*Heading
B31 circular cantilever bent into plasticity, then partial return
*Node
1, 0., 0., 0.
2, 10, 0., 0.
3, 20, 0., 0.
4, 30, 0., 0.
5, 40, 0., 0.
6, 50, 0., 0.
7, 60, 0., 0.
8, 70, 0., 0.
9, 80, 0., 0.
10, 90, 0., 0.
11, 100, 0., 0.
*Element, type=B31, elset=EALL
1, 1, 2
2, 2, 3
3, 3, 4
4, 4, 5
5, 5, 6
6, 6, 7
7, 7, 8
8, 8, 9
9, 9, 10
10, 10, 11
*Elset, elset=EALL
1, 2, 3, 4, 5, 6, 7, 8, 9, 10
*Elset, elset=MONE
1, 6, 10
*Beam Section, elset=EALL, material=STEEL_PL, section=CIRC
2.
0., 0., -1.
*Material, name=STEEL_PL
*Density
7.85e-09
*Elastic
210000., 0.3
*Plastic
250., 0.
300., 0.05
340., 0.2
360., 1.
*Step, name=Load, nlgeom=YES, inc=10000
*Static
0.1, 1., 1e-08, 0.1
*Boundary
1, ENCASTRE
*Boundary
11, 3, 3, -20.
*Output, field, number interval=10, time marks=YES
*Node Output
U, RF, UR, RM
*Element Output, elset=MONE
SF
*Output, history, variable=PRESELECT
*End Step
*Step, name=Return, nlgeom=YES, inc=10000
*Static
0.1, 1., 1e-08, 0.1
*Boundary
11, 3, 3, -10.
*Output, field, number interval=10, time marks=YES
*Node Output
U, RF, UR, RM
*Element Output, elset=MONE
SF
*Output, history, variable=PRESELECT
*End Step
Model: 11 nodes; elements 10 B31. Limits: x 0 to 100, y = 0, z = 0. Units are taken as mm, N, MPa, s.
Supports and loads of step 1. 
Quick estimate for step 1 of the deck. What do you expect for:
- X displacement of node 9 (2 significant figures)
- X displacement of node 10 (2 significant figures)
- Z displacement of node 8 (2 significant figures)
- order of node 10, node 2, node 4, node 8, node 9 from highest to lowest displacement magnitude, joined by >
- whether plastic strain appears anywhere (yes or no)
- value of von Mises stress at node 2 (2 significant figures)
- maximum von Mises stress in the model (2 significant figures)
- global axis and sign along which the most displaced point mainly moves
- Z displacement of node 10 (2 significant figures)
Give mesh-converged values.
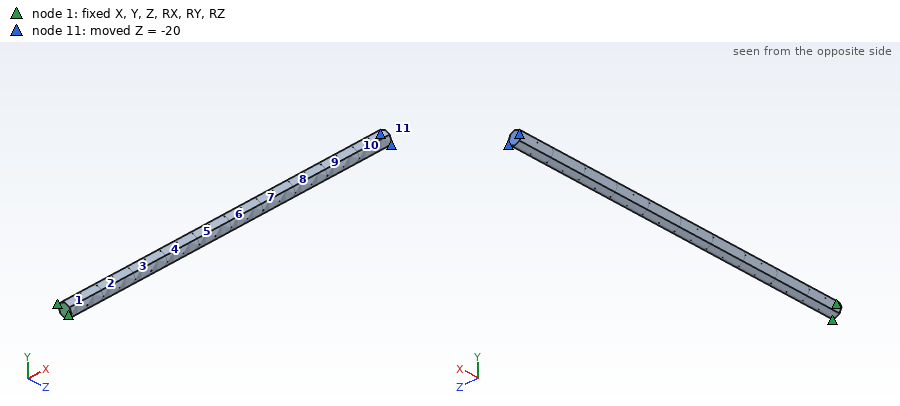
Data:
-1.3 mm
-1.6 mm
-13 mm
node 10 > node 9 > node 8 > node 4 > node 2
yes
380 MPa
420 MPa
-Z
-18 mm
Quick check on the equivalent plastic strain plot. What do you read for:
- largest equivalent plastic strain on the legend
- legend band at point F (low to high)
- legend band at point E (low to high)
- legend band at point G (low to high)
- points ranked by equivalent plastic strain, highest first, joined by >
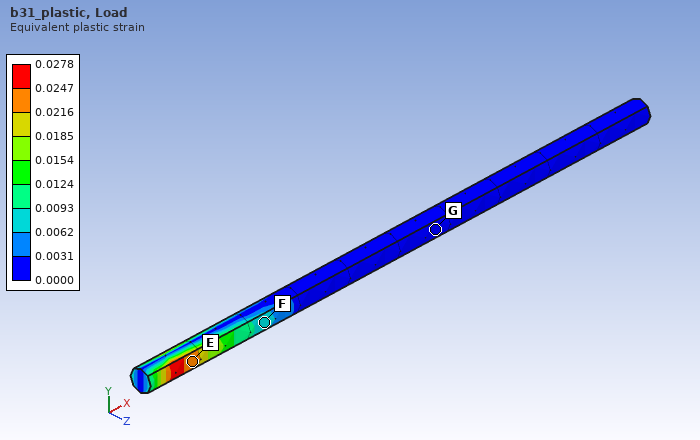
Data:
0.0278
0.0062 to 0.0093
0.0216 to 0.0247
0.0000 to 0.0031
E > F > G
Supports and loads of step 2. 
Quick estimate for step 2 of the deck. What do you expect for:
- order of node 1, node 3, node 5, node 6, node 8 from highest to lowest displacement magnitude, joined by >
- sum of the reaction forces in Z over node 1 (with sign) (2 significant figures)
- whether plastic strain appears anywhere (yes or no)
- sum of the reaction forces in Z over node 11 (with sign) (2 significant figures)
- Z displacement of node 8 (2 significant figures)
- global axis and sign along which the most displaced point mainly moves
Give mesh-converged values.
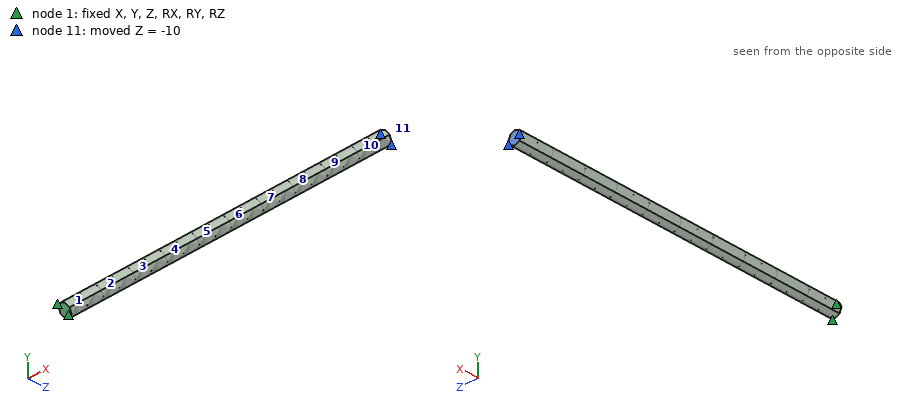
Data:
node 8 > node 6 > node 5 > node 3 > node 1
-22 N
yes
21 N
-6.8 mm
-Z
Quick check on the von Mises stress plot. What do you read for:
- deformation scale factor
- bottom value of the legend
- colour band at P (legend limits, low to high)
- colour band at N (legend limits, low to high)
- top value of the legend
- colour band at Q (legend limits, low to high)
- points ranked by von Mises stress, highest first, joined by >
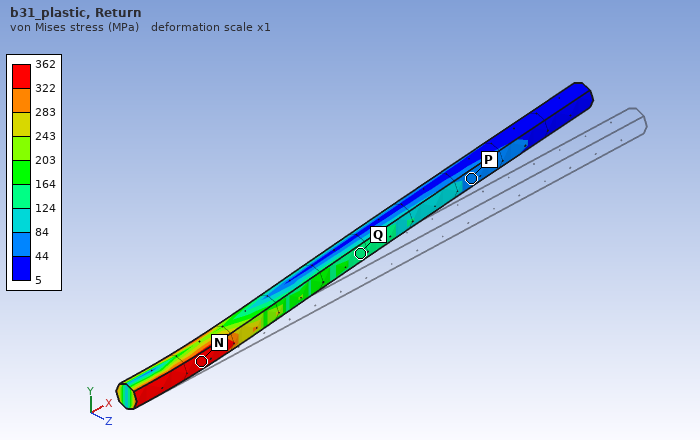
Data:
1
5 MPa
44 to 84 MPa
322 to 362 MPa
362 MPa
124 to 164 MPa
N > Q > P
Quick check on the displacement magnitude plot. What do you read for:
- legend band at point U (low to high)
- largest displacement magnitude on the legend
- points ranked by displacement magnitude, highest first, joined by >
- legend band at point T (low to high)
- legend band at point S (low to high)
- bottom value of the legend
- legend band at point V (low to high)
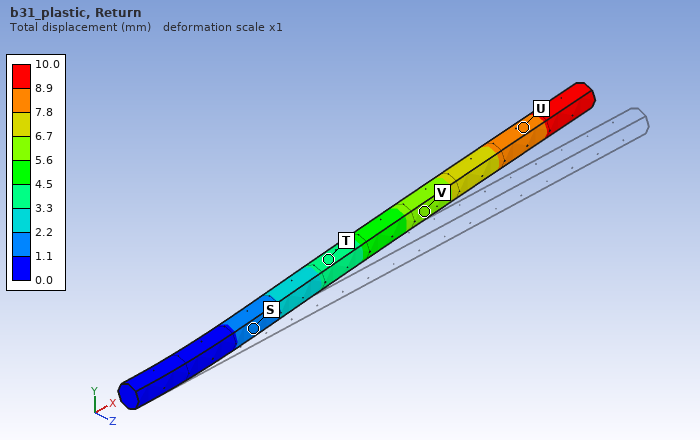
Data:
7.8 to 8.9 mm
10.0 mm
U > V > T > S
3.3 to 4.5 mm
1.1 to 2.2 mm
0.0 mm
5.6 to 6.7 mm
